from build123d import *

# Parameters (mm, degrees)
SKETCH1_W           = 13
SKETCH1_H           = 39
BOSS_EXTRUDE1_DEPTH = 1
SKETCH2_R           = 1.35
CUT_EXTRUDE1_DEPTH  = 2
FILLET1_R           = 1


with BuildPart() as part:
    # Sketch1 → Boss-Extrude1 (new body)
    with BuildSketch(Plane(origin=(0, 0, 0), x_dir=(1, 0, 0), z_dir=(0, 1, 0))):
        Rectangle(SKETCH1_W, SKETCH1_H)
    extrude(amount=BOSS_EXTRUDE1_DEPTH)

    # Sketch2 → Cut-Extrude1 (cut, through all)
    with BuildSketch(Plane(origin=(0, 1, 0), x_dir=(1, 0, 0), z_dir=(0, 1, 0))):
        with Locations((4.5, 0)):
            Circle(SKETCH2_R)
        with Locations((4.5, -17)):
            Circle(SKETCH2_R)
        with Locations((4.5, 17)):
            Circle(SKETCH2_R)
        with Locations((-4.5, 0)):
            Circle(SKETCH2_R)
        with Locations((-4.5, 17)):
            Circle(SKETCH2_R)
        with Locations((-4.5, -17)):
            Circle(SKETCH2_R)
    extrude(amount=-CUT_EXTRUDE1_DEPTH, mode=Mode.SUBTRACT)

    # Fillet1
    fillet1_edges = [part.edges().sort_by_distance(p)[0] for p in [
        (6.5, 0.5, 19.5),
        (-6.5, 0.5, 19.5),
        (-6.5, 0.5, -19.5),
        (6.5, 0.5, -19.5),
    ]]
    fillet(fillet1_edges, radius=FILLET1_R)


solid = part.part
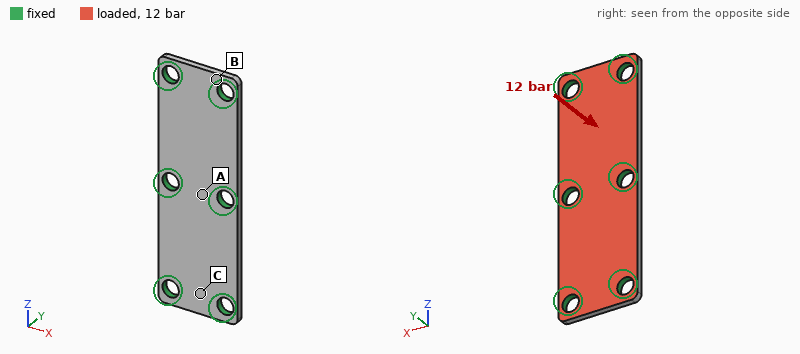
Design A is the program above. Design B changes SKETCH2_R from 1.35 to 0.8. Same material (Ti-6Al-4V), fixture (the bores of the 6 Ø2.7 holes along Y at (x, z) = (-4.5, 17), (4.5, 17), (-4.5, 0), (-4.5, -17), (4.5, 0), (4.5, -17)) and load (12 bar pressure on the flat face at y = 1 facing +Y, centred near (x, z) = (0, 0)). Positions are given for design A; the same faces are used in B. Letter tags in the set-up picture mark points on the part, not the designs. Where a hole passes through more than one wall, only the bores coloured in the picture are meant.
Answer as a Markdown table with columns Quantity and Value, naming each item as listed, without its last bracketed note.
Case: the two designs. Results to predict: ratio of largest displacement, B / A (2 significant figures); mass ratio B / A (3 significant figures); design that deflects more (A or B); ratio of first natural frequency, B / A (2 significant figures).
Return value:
| Quantity | Value |
|---|---|
| ratio of largest displacement, B / A | 1.4 |
| mass ratio B / A | 1.05 |
| design that deflects more | B |
| ratio of first natural frequency, B / A | 0.83 |
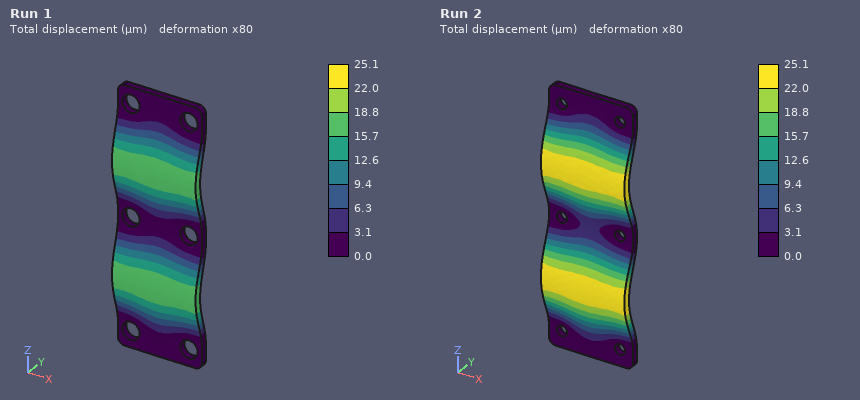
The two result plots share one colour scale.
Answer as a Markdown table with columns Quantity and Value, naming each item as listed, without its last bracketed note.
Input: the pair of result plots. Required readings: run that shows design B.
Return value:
| Quantity | Value |
|---|---|
| run that shows design B | Run 2 |
